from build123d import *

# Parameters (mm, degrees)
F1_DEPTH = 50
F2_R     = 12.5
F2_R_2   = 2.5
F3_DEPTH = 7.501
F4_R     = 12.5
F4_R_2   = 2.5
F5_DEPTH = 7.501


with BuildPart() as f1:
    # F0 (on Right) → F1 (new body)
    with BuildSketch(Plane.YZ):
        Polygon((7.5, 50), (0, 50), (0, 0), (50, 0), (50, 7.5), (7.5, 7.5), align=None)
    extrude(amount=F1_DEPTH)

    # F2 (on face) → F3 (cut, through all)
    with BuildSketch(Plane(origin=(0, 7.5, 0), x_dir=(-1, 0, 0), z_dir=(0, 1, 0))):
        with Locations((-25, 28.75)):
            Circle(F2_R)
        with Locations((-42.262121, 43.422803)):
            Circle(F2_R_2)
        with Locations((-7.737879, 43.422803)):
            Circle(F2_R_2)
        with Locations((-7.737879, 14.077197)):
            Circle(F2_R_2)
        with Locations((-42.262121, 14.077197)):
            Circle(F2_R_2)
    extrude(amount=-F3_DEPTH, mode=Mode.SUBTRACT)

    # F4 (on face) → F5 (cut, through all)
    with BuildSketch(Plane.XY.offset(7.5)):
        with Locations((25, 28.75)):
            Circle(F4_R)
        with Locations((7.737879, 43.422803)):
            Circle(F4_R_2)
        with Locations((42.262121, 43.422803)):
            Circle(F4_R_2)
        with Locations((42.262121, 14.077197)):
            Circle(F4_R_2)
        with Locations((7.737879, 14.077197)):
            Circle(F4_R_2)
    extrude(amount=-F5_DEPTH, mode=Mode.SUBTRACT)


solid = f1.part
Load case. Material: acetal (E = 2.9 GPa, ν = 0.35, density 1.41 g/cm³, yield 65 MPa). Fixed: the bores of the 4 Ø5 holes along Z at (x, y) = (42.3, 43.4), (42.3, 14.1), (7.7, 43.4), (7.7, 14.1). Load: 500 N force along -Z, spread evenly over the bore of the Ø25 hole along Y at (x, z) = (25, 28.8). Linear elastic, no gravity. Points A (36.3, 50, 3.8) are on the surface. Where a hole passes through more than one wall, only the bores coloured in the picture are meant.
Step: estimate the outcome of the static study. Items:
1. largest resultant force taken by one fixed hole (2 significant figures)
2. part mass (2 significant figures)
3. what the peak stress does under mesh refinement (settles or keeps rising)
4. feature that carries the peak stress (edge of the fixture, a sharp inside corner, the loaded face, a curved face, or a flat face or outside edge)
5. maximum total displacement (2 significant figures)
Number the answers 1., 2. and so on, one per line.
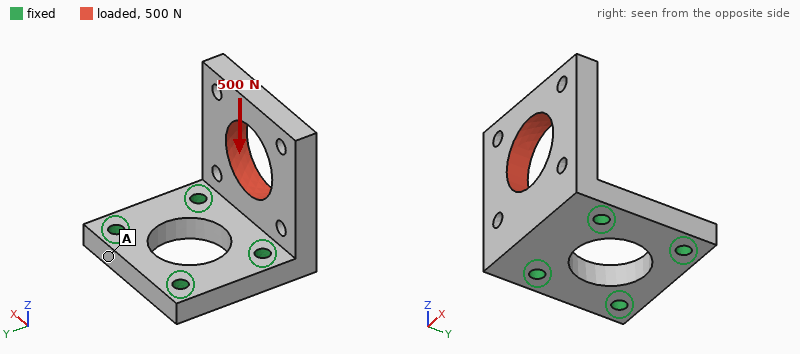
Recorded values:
1. 260 N
2. 37 g
3. keeps rising
4. edge of the fixture
5. 0.34 mm
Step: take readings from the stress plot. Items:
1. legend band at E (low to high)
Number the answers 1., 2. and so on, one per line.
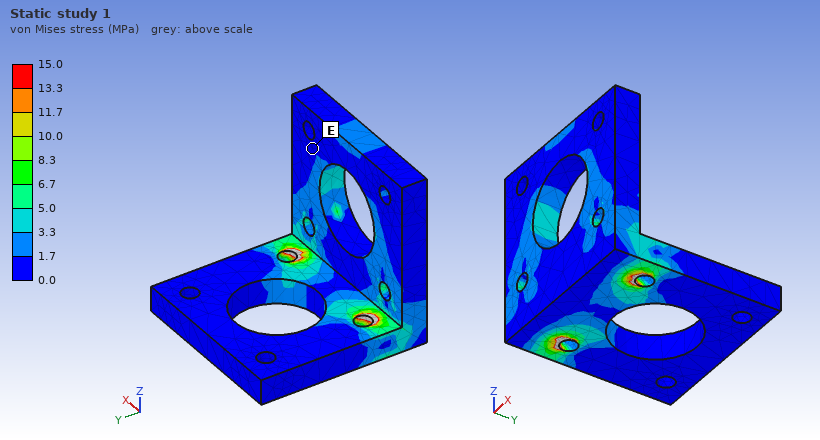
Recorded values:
1. 0.0 to 1.7 MPa
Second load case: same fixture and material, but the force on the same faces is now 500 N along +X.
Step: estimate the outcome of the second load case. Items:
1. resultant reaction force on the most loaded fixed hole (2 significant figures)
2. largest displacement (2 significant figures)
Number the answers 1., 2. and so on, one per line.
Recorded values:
1. 430 N
2. 0.36 mm
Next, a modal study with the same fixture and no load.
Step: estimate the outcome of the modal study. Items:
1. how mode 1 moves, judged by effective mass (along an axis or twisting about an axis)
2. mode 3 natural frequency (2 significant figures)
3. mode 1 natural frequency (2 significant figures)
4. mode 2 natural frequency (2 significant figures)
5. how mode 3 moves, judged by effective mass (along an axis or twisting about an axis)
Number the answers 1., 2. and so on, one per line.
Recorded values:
1. along Y
2. 1800 Hz
3. 600 Hz
4. 1300 Hz
5. along X
